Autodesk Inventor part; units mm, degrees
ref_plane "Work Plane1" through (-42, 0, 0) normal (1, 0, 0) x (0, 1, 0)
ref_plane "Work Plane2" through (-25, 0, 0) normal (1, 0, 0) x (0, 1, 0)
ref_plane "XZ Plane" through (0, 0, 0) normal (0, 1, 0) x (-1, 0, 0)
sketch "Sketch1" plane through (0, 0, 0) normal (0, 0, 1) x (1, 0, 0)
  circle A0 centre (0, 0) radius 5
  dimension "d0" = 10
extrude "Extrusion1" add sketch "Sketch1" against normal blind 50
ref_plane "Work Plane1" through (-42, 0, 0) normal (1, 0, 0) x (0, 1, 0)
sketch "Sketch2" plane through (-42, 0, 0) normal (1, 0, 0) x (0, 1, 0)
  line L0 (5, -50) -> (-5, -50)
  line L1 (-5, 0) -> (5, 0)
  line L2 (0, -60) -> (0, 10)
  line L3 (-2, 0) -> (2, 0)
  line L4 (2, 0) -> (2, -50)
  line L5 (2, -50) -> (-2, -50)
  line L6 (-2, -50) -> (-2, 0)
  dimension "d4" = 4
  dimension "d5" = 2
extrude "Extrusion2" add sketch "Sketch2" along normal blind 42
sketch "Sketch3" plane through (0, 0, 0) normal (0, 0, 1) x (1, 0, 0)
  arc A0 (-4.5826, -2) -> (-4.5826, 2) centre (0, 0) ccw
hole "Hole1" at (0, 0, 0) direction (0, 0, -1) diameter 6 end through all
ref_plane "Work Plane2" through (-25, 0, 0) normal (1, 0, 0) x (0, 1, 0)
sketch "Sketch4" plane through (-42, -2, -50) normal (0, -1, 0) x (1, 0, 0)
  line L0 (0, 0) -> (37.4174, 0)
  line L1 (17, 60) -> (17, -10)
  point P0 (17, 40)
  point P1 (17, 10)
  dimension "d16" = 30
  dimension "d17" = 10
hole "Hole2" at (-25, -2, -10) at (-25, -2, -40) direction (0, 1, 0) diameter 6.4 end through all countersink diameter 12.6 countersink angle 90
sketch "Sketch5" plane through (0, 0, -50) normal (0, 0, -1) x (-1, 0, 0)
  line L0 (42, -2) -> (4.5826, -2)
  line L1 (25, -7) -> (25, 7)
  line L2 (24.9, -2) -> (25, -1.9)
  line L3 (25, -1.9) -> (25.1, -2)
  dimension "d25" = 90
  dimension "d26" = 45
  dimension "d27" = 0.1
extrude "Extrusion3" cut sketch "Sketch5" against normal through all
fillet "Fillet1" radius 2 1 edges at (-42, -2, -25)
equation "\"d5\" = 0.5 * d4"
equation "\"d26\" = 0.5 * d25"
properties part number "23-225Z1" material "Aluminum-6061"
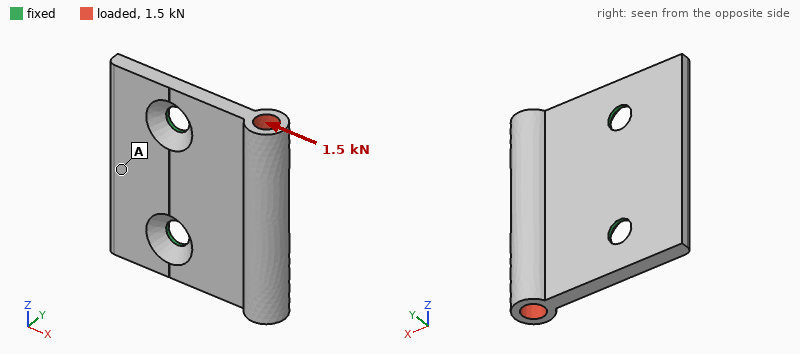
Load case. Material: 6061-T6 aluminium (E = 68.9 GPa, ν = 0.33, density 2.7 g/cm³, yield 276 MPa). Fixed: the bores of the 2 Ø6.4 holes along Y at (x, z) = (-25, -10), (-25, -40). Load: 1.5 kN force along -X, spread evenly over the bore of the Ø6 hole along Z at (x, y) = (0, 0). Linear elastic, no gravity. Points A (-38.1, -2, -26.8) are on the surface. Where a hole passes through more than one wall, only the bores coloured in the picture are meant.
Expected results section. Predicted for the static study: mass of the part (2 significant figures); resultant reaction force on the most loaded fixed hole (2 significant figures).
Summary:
25 g
750 N
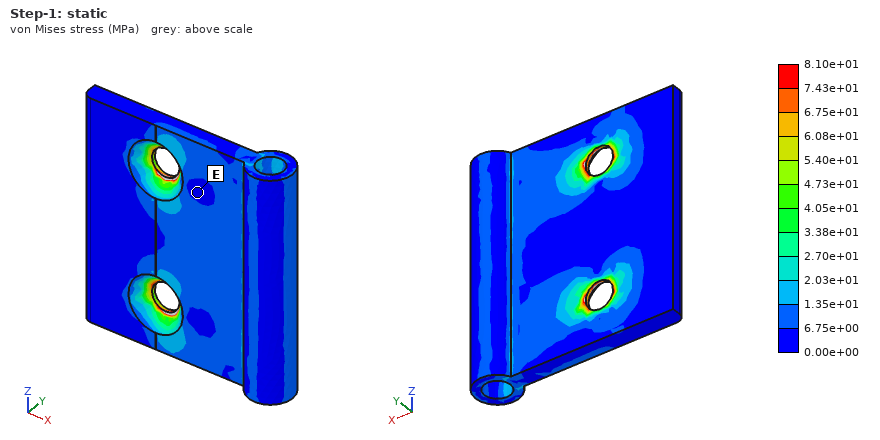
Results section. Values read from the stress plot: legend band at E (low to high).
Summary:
0.00e+00 to 6.75e+00 MPa
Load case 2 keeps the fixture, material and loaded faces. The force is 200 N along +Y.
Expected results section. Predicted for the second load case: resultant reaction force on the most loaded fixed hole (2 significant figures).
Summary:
120 N
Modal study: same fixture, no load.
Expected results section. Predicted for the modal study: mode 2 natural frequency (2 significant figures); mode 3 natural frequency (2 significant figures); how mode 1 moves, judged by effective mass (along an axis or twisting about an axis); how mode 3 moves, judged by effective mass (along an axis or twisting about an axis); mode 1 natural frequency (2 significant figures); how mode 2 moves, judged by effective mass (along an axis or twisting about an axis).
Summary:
5400 Hz
7700 Hz
along Y
along Y
2200 Hz
twisting about X
